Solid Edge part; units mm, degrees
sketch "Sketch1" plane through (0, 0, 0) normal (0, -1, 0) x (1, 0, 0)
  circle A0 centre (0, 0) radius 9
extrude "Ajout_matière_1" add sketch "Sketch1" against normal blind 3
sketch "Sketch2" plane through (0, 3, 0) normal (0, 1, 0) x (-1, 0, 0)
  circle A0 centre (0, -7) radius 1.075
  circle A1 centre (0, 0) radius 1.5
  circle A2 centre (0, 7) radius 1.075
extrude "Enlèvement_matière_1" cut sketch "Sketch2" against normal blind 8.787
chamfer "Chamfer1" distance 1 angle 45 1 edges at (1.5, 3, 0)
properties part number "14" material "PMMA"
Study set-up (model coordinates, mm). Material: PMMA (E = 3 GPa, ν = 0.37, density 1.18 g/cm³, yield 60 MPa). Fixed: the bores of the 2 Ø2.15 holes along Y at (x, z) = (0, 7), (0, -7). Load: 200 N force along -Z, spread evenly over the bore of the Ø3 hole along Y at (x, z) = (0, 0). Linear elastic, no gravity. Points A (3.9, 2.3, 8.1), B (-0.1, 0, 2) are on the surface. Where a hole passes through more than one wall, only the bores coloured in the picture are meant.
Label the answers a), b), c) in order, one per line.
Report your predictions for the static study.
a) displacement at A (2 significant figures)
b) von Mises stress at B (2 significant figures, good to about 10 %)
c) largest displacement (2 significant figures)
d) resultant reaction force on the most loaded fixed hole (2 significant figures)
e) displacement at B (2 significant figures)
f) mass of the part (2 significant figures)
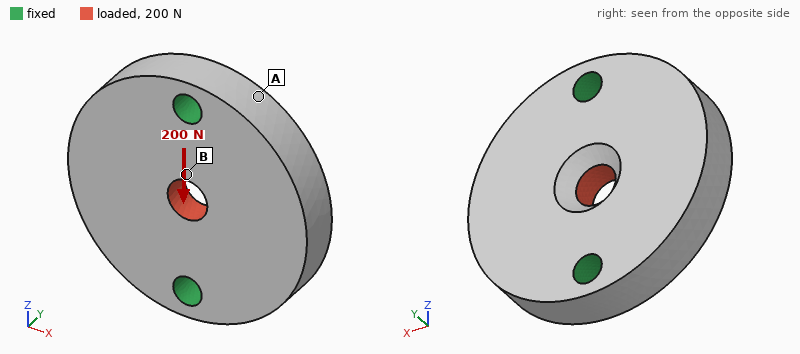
a) 5.6 µm
b) 12 MPa
c) 16 µm
d) 100 N
e) 14 µm
f) 0.84 g
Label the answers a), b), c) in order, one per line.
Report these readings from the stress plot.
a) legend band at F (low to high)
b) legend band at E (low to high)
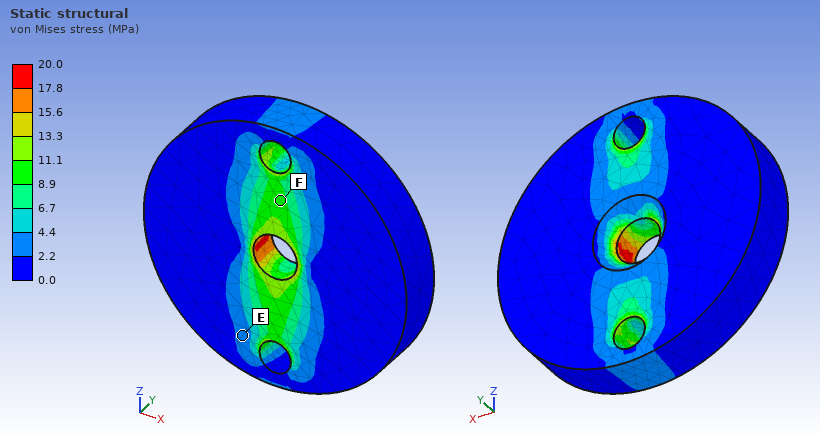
a) 8.9 to 11.1 MPa
b) 2.2 to 4.4 MPa
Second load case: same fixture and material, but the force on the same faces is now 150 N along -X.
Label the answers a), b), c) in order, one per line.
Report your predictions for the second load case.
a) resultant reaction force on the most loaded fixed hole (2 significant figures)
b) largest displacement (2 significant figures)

a) 75 N
b) 20 µm
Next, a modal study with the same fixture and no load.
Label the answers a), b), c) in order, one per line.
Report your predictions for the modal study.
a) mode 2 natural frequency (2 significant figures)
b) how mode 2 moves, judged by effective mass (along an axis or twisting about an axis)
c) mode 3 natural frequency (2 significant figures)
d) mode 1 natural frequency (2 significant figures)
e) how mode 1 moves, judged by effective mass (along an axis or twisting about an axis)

a) 10 kHz
b) along Y
c) 21 kHz
d) 8500 Hz
e) twisting about Z
